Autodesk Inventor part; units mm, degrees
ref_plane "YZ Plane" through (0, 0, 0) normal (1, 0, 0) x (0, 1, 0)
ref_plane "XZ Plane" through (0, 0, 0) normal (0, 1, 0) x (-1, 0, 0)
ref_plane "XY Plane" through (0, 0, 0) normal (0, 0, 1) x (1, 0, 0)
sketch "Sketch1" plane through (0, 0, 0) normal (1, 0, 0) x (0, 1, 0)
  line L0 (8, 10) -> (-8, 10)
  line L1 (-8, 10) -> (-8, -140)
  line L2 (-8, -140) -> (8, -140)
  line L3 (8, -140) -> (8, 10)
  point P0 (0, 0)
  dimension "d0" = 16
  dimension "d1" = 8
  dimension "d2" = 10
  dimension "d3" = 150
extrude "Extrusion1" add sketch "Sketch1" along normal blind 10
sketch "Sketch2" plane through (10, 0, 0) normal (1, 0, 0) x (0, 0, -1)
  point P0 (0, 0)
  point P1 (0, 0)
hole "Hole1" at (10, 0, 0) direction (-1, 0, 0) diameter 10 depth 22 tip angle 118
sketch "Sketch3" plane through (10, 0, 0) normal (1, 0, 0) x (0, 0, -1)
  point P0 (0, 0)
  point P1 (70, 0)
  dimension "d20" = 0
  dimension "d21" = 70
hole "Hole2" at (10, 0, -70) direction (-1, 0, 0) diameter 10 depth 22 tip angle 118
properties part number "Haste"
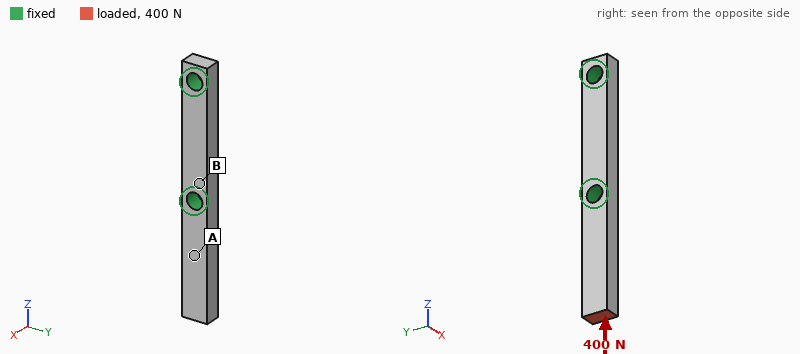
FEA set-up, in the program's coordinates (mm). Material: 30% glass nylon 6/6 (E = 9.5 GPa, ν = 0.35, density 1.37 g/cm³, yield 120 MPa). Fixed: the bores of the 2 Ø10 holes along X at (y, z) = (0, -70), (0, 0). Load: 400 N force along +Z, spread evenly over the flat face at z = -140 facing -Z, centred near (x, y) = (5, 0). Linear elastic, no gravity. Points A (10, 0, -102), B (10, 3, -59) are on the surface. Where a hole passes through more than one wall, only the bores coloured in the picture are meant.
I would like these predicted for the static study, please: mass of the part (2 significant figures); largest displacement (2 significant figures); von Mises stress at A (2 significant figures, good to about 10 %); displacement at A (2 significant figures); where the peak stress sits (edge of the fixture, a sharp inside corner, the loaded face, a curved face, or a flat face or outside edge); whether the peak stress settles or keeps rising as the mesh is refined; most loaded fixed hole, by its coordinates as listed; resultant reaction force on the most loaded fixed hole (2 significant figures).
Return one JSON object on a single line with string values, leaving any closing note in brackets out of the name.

{"mass of the part": "31 g", "largest displacement": "18 µm", "von Mises stress at A": "2.5 MPa", "displacement at A": "7.6 µm", "where the peak stress sits": "edge of the fixture", "whether the peak stress settles or keeps rising as the mesh is refined": "keeps rising", "most loaded fixed hole, by its coordinates as listed": "(0, -70)", "resultant reaction force on the most loaded fixed hole": "400 N"}
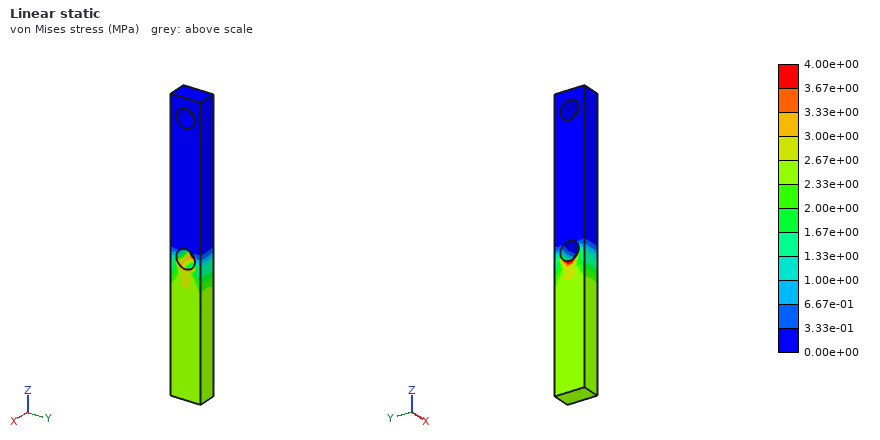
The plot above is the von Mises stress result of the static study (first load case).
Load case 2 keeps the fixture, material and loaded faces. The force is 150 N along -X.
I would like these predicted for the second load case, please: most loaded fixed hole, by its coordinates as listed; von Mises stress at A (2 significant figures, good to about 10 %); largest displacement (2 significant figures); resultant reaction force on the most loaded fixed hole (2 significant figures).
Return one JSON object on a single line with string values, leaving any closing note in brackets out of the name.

{"most loaded fixed hole, by its coordinates as listed": "(0, -70)", "von Mises stress at A": "21 MPa", "largest displacement": "1.2 mm", "resultant reaction force on the most loaded fixed hole": "150 N"}
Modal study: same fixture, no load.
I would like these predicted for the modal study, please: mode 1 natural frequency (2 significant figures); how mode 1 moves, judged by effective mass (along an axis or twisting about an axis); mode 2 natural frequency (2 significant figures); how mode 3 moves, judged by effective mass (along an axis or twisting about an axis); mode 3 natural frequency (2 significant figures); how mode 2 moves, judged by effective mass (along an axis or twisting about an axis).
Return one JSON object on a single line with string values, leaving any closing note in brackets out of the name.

{"mode 1 natural frequency": "950 Hz", "how mode 1 moves, judged by effective mass": "along X", "mode 2 natural frequency": "1400 Hz", "how mode 3 moves, judged by effective mass": "twisting about Z", "mode 3 natural frequency": "5100 Hz", "how mode 2 moves, judged by effective mass": "along Y"}
